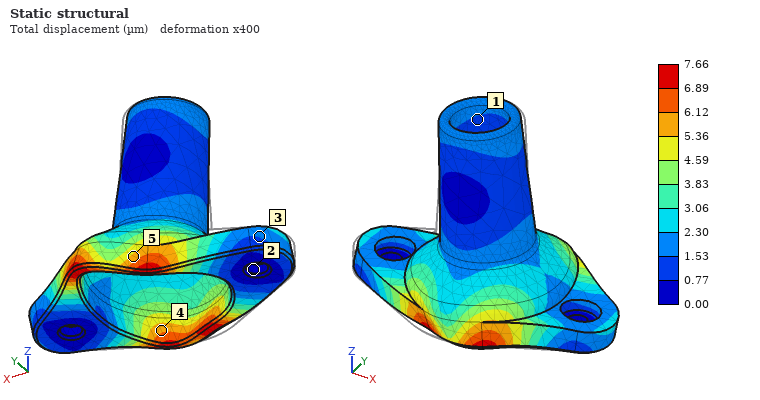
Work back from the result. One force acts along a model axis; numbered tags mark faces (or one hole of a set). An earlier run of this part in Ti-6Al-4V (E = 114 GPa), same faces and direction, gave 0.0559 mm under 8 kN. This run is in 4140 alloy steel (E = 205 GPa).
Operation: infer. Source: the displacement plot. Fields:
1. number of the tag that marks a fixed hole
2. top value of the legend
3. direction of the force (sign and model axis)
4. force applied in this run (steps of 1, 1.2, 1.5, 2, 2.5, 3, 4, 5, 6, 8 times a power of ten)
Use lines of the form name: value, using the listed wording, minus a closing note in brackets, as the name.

number of the tag that marks a fixed hole: 2
top value of the legend: 7.66 µm
direction of the force: +X
force applied in this run: 2 kN
